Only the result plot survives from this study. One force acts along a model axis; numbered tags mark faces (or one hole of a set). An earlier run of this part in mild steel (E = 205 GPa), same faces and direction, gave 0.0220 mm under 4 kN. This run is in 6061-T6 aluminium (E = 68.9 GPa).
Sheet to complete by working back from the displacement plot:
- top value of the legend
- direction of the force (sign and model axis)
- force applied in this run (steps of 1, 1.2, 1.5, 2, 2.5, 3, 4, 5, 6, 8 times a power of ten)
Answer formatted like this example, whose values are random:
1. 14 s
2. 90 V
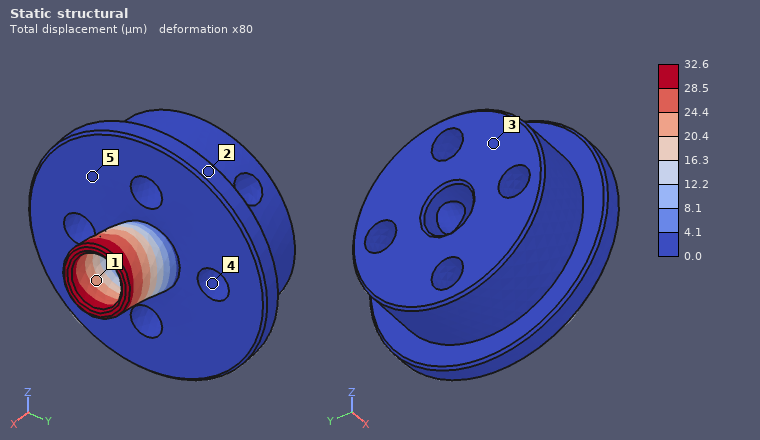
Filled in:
1. 32.6 µm
2. +Z
3. 2 kN
